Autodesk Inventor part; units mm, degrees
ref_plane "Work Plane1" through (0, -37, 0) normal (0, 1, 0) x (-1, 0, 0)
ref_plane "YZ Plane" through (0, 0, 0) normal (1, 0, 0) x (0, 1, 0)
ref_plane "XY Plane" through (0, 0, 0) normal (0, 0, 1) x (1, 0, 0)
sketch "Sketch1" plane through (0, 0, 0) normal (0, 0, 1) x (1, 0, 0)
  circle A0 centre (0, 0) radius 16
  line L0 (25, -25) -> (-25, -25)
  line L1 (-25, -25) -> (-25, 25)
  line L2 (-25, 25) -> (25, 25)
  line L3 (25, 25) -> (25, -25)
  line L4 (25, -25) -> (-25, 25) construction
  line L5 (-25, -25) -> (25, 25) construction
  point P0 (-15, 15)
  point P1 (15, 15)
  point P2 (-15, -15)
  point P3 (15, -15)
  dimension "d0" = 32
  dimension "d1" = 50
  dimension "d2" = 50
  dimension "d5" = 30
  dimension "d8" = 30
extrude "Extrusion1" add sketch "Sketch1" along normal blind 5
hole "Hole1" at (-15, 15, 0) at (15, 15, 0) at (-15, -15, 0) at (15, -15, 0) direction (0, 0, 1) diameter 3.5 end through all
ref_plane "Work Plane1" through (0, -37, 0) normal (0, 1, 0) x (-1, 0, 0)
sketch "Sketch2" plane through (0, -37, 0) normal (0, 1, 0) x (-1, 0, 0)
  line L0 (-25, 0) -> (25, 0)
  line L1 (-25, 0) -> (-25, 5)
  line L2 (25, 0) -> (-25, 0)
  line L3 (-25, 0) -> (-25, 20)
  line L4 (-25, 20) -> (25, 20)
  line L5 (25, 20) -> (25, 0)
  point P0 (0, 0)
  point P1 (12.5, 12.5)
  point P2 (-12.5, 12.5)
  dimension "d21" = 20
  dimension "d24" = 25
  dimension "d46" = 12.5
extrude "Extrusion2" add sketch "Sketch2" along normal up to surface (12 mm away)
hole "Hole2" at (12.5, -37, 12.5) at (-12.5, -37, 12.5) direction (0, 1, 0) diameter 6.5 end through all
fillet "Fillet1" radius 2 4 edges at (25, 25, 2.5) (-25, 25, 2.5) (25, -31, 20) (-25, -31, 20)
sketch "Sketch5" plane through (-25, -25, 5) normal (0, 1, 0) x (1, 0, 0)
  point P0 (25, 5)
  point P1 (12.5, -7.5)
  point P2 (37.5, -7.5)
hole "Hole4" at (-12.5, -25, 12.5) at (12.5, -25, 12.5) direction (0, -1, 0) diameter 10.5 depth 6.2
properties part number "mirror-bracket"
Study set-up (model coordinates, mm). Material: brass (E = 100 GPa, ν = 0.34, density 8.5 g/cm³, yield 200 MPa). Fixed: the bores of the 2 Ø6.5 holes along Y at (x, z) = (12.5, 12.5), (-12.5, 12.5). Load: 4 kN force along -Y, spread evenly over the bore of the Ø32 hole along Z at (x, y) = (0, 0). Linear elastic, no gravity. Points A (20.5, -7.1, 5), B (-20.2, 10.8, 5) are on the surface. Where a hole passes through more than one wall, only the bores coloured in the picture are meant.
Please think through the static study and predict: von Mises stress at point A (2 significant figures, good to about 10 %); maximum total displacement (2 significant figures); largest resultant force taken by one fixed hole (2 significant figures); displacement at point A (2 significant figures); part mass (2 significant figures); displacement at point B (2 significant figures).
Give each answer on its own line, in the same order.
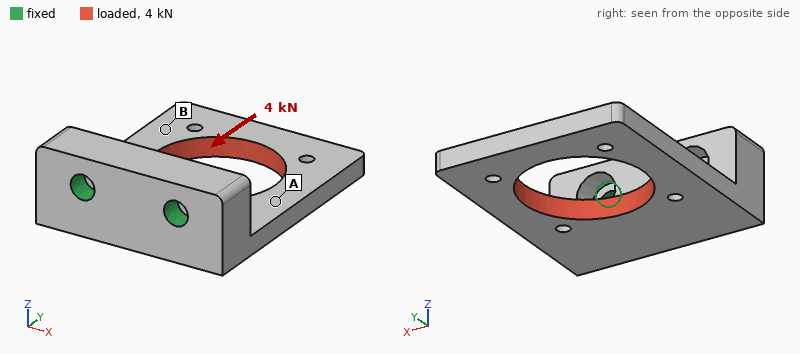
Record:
28 MPa
83 µm
2.0 kN
38 µm
160 g
59 µm
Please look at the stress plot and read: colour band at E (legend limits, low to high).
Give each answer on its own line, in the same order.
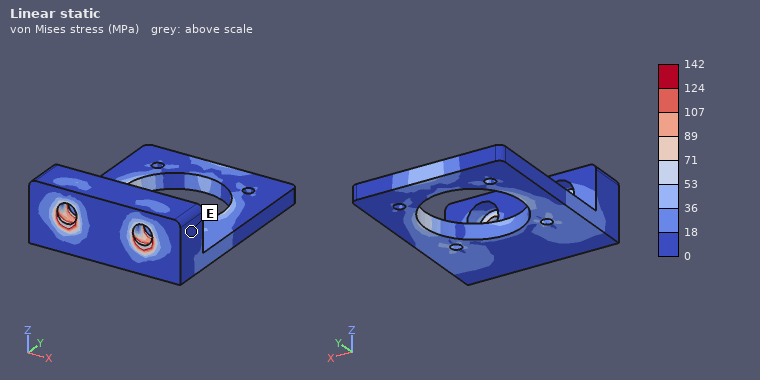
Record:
0 to 18 MPa
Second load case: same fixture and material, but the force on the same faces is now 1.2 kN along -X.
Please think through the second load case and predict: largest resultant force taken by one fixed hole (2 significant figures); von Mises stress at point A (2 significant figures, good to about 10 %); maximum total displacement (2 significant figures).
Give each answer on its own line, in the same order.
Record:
1.6 kN
19 MPa
55 µm
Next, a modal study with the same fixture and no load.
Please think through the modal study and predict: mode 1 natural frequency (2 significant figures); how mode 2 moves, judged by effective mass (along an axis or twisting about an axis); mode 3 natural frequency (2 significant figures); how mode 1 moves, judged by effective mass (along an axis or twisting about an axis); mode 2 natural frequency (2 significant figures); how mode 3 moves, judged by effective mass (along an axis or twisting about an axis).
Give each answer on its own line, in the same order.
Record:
840 Hz
twisting about Y
3200 Hz
along Z
1900 Hz
along X
